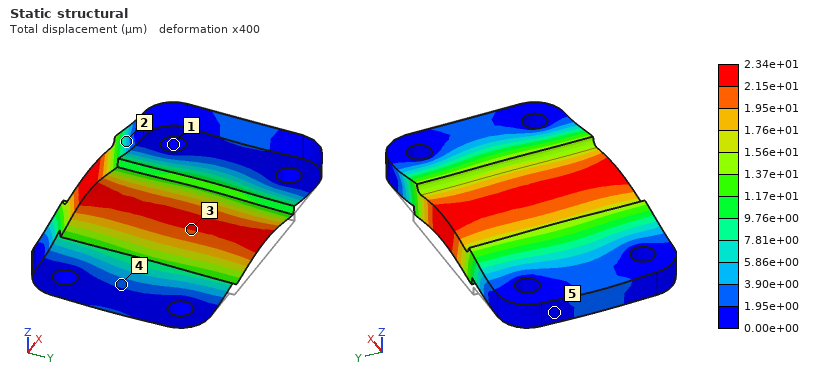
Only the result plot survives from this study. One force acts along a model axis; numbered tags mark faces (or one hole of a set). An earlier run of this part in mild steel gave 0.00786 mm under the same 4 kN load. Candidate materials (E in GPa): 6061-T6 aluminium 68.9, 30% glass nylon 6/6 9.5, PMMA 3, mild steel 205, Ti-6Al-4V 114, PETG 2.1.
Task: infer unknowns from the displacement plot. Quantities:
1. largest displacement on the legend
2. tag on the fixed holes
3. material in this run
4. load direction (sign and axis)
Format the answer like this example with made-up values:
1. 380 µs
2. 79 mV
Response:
1. 2.34e+01 µm
2. 1
3. 6061-T6 aluminium
4. +Z
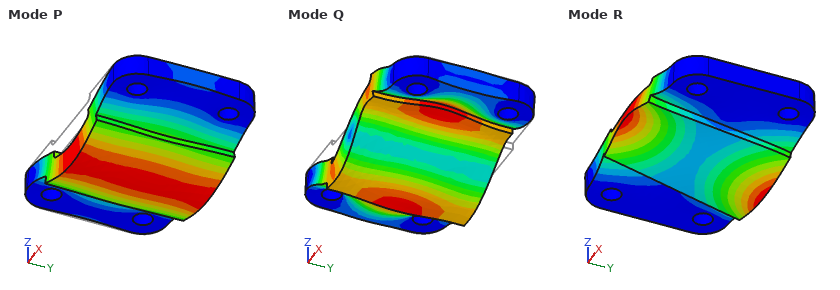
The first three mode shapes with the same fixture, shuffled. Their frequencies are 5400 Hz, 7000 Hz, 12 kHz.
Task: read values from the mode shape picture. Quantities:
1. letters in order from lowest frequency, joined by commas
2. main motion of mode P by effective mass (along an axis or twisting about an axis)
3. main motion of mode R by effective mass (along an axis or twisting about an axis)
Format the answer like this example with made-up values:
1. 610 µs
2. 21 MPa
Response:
1. P, R, Q
2. along Z
3. twisting about X
